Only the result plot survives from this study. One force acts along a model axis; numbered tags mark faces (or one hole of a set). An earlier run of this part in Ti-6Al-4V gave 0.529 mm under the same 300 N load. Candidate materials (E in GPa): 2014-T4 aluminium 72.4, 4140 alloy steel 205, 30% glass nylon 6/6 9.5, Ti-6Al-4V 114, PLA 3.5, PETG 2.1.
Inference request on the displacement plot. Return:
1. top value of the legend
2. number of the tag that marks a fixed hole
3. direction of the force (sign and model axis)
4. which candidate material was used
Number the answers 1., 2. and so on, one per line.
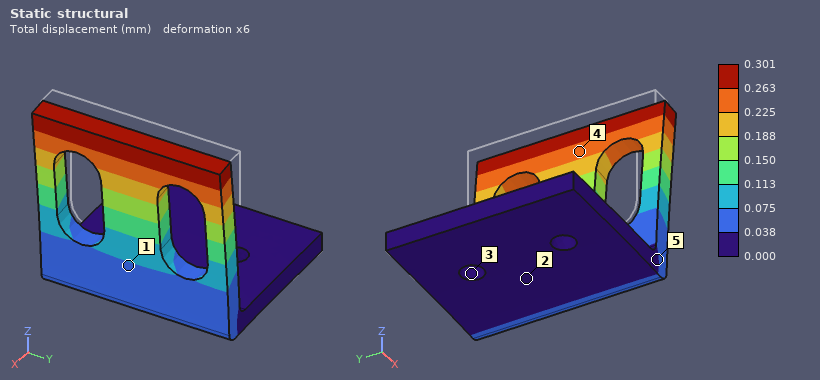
1. 0.301 mm
2. 3
3. +X
4. 4140 alloy steel
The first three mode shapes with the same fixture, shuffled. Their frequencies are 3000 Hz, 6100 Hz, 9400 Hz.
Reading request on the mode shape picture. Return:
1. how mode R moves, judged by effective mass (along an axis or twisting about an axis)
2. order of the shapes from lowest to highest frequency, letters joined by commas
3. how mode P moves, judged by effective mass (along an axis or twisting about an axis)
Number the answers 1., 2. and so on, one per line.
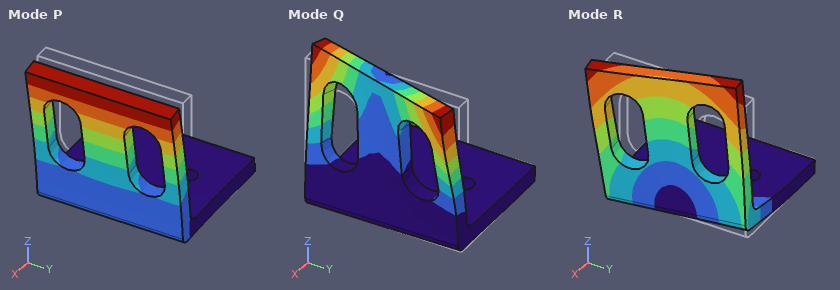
1. along Y
2. P, R, Q
3. along X
